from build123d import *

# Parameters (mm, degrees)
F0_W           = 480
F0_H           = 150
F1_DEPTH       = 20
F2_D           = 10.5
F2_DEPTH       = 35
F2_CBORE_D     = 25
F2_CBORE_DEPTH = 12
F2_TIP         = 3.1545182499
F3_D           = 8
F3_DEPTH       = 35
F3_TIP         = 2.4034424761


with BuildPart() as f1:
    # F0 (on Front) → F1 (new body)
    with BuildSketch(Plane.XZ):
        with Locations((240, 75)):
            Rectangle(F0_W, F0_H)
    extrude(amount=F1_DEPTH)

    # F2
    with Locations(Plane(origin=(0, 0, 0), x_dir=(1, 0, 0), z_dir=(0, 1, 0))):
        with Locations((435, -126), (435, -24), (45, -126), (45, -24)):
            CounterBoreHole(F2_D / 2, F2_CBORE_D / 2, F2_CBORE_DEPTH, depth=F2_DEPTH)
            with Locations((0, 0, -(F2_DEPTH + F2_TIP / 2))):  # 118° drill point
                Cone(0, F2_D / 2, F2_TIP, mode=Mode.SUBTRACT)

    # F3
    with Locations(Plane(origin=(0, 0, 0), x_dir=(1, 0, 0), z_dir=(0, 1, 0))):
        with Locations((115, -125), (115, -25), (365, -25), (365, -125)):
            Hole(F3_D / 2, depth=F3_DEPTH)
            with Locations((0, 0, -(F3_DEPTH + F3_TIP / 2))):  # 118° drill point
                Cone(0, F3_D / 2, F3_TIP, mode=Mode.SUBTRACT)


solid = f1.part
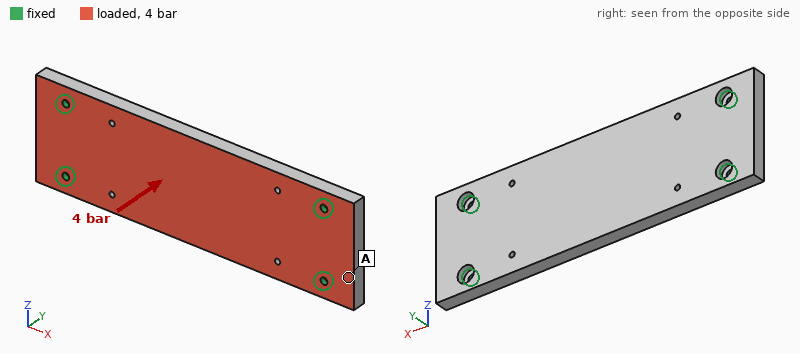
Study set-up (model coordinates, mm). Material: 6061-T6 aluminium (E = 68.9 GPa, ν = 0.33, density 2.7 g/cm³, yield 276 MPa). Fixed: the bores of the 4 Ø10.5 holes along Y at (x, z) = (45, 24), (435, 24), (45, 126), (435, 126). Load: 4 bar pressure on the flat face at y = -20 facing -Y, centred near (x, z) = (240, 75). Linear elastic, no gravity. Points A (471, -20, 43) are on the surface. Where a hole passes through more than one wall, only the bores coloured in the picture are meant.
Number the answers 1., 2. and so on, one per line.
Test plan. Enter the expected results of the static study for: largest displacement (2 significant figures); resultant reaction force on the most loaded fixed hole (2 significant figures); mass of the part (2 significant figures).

1. 1.0 mm
2. 15 kN
3. 3.8 kg
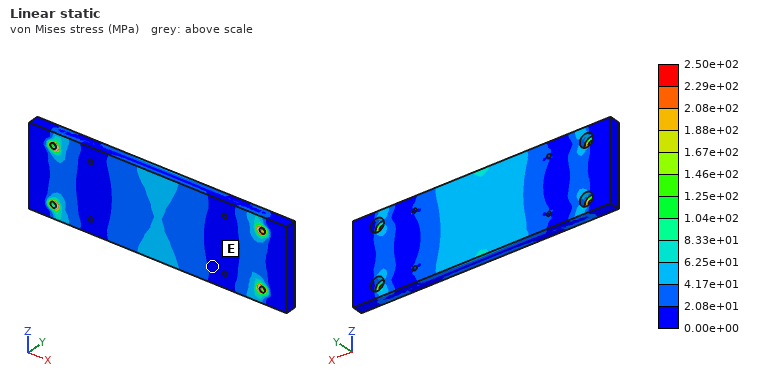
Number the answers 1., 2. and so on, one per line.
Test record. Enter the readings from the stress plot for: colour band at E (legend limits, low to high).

1. 0.00e+00 to 2.08e+01 MPa
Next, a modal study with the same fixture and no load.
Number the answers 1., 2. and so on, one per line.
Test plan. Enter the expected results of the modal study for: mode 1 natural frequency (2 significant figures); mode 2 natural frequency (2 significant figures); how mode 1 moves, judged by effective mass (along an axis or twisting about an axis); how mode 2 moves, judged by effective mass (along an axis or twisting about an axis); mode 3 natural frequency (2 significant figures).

1. 490 Hz
2. 1100 Hz
3. along Y
4. twisting about X
5. 1400 Hz
